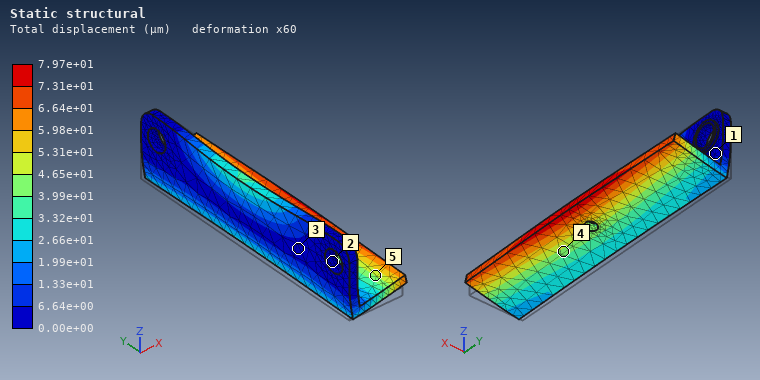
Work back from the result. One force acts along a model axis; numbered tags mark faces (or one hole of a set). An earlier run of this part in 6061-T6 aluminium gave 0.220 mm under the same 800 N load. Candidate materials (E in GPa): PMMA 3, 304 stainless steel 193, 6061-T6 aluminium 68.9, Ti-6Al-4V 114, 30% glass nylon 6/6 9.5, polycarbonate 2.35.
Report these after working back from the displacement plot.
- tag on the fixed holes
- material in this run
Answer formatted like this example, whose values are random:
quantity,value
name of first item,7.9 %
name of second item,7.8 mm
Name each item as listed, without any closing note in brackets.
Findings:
quantity,value
tag on the fixed holes,2
material in this run,304 stainless steel
